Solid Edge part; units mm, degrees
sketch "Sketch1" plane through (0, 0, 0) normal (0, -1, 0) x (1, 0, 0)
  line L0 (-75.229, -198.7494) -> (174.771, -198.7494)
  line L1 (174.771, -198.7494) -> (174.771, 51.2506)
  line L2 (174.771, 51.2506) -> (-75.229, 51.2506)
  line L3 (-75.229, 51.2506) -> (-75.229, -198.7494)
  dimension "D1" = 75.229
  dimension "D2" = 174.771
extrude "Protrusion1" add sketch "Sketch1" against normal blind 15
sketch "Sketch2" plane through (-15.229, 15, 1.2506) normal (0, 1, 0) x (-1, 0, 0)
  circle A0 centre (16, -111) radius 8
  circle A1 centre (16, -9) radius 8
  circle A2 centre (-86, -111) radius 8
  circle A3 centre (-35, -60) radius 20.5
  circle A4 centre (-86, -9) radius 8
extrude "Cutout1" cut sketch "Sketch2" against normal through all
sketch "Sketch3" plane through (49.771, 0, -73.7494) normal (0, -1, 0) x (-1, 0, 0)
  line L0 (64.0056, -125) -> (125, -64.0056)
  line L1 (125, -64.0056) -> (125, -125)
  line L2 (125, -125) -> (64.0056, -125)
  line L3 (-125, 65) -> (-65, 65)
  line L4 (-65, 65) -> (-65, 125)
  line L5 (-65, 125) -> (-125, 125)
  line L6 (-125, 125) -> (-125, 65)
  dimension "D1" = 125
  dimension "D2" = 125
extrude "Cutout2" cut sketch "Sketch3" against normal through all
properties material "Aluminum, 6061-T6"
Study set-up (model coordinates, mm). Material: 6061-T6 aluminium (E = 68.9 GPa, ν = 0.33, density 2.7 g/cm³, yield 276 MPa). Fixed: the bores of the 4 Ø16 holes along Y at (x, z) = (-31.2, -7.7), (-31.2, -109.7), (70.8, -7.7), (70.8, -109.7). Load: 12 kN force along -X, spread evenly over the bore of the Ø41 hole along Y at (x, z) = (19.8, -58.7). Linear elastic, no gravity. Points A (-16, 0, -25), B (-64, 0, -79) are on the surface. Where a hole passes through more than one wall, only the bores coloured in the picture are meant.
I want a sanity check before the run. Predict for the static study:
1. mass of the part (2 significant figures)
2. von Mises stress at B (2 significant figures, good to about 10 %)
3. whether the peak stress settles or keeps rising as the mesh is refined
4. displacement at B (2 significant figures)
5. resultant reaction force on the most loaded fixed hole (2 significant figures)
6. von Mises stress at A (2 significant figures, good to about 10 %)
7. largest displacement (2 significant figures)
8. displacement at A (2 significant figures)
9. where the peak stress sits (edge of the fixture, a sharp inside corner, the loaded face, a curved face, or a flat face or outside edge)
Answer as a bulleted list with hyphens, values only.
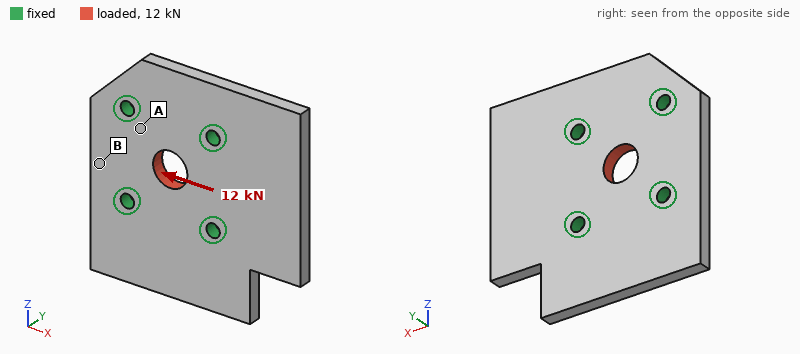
- 2.2 kg
- 1.9 MPa
- keeps rising
- 2.2 µm
- 3.2 kN
- 5.5 MPa
- 5.3 µm
- 1.7 µm
- edge of the fixture
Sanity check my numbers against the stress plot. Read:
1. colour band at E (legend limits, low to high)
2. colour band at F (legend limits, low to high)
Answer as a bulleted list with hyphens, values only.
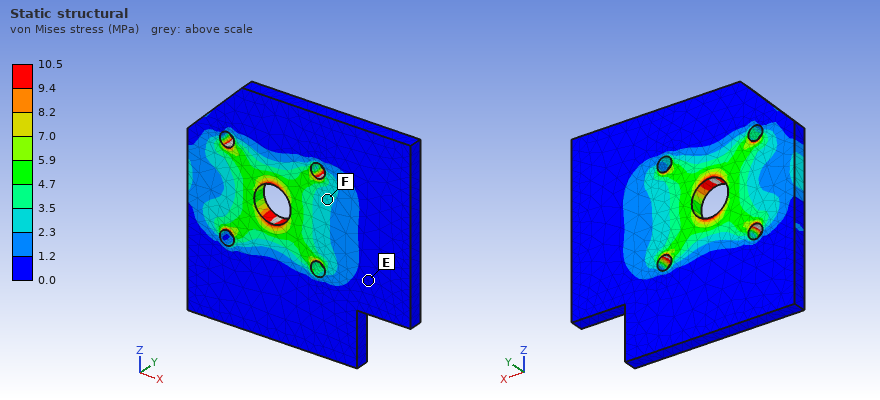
- 0.0 to 1.2 MPa
- 2.3 to 3.5 MPa
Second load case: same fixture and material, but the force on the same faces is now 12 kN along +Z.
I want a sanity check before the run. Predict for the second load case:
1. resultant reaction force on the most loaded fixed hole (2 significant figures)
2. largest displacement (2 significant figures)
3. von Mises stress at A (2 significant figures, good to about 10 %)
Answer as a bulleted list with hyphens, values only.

- 3.2 kN
- 5.1 µm
- 5.3 MPa
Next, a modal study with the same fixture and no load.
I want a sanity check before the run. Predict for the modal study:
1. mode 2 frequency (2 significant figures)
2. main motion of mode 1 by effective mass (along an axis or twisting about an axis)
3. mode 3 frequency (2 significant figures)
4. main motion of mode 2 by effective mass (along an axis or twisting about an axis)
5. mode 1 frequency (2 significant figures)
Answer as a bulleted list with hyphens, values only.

- 1500 Hz
- along Y
- 1700 Hz
- along Y
- 1100 Hz
